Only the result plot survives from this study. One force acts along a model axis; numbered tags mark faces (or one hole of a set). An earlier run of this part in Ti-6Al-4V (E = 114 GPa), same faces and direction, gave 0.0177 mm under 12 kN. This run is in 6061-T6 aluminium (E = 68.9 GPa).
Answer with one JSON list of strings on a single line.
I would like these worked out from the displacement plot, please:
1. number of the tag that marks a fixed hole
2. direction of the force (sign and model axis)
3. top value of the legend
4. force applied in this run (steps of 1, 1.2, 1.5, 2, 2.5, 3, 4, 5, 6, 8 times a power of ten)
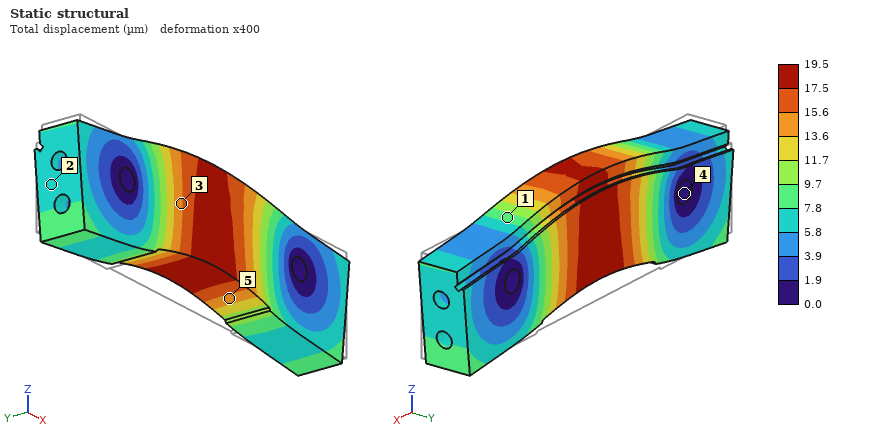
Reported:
["4", "+Z", "19.5 µm", "8 kN"]
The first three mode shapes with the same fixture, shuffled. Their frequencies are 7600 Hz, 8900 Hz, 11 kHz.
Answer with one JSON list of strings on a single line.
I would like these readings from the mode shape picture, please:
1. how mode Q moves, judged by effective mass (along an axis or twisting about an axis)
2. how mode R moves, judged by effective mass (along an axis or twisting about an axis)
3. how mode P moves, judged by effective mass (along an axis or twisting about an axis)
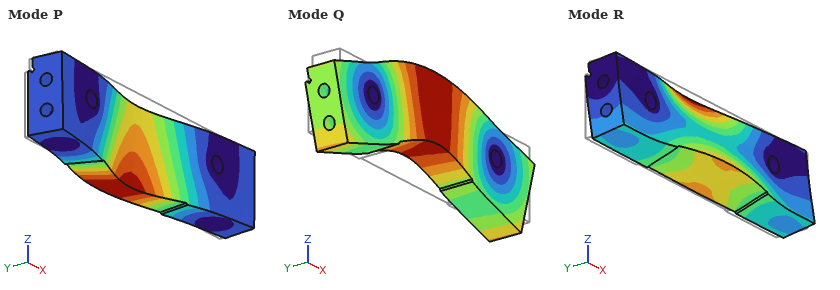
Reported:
["along Z", "twisting about X", "along Y"]
